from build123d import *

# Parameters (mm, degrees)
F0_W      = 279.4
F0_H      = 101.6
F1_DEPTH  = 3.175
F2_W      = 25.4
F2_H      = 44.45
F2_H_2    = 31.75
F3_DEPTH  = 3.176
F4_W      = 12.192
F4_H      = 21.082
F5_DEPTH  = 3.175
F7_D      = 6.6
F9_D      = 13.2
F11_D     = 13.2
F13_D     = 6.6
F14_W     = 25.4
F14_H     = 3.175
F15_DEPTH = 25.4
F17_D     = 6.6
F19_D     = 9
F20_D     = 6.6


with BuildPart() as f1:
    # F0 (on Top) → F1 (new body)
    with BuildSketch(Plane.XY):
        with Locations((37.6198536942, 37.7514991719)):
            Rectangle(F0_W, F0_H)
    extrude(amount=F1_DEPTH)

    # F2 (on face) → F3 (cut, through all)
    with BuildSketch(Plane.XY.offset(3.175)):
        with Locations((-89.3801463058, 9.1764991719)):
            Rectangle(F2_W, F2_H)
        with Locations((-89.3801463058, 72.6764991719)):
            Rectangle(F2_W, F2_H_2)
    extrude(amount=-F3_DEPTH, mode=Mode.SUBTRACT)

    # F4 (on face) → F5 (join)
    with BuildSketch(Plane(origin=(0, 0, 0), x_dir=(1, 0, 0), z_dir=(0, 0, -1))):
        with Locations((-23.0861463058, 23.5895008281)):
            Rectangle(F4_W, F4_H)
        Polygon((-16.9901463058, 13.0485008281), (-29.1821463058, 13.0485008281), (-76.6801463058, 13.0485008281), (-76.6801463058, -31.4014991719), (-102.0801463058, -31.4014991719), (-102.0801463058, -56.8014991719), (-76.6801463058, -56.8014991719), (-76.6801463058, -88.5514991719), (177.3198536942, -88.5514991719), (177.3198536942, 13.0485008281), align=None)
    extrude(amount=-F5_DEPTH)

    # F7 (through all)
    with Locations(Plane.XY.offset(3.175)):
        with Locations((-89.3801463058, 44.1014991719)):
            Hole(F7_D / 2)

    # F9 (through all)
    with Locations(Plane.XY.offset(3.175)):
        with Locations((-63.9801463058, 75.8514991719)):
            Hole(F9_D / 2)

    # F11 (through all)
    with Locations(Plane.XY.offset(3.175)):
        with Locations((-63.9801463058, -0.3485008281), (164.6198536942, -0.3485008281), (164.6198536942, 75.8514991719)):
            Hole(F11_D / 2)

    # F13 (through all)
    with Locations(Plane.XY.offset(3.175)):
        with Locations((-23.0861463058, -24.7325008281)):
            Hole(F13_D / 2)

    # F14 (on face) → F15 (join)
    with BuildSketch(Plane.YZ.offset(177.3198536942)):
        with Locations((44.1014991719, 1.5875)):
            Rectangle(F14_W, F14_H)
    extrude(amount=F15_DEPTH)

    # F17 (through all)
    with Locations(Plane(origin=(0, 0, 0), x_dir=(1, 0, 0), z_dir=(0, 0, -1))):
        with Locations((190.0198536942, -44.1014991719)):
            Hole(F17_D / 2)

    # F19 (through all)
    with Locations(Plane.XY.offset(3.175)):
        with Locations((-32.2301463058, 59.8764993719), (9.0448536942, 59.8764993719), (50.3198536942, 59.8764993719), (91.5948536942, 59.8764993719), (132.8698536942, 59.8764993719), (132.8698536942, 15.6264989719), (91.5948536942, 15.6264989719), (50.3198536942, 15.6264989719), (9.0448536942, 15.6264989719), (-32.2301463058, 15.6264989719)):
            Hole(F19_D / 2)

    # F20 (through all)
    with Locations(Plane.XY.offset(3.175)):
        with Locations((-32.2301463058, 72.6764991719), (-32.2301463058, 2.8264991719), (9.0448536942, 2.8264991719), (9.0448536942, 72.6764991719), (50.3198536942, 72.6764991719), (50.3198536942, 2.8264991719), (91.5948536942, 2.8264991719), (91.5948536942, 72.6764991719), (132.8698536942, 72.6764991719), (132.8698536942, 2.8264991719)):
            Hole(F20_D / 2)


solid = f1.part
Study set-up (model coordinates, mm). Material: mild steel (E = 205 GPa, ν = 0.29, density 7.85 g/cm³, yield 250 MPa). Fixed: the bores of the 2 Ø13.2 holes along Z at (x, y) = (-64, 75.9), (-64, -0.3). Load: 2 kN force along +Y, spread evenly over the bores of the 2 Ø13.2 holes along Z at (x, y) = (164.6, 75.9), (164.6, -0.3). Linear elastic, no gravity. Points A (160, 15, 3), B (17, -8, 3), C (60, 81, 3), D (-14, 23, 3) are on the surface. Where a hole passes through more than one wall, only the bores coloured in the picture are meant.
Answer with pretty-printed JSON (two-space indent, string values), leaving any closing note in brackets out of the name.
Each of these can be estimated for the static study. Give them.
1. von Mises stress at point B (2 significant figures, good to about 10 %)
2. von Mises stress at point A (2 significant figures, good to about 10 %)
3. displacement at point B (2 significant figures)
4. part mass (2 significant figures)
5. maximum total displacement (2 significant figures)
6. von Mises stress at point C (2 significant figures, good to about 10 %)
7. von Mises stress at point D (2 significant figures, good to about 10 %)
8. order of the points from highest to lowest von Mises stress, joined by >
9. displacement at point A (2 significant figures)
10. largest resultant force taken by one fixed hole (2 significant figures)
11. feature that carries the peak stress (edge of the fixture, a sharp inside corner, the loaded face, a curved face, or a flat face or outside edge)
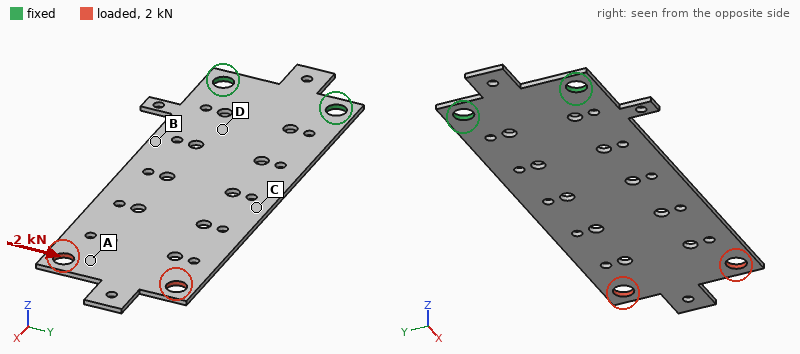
{
  "von Mises stress at point B": "56 MPa",
  "von Mises stress at point A": "10 MPa",
  "displacement at point B": "0.043 mm",
  "part mass": "640 g",
  "maximum total displacement": "0.22 mm",
  "von Mises stress at point C": "38 MPa",
  "von Mises stress at point D": "21 MPa",
  "order of the points from highest to lowest von Mises stress, joined by >": "B > C > D > A",
  "displacement at point A": "0.17 mm",
  "largest resultant force taken by one fixed hole": "5.8 kN",
  "feature that carries the peak stress": "a curved face"
}
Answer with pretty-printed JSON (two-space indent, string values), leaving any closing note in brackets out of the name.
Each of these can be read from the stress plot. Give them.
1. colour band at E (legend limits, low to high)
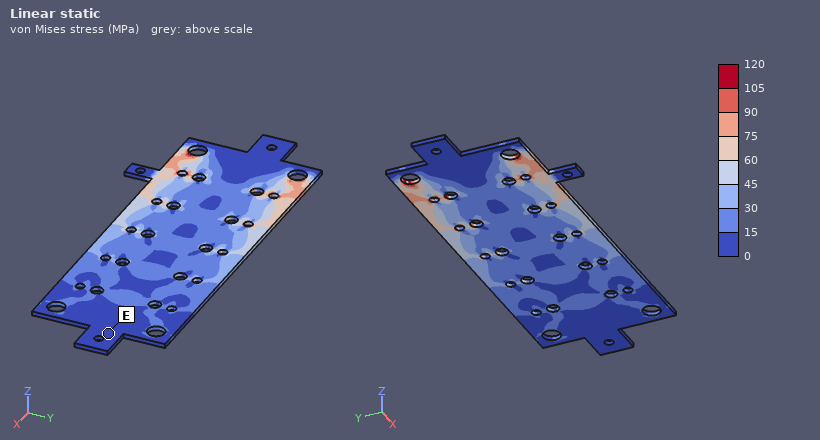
{
  "colour band at E": "0 to 15 MPa"
}
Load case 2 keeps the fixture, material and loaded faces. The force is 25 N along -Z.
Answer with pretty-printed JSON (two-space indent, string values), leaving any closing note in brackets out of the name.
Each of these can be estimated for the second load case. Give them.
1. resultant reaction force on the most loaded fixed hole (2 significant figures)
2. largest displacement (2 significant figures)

{
  "resultant reaction force on the most loaded fixed hole": "13 N",
  "largest displacement": "2.4 mm"
}
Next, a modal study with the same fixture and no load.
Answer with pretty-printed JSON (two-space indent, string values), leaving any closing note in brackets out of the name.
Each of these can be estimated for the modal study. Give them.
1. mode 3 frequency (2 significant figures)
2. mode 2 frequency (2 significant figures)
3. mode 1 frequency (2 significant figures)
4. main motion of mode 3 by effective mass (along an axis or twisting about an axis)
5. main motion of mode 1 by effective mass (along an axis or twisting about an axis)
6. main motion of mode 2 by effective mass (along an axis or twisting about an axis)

{
  "mode 3 frequency": "260 Hz",
  "mode 2 frequency": "230 Hz",
  "mode 1 frequency": "43 Hz",
  "main motion of mode 3 by effective mass": "along Z",
  "main motion of mode 1 by effective mass": "along Z",
  "main motion of mode 2 by effective mass": "twisting about X"
}
